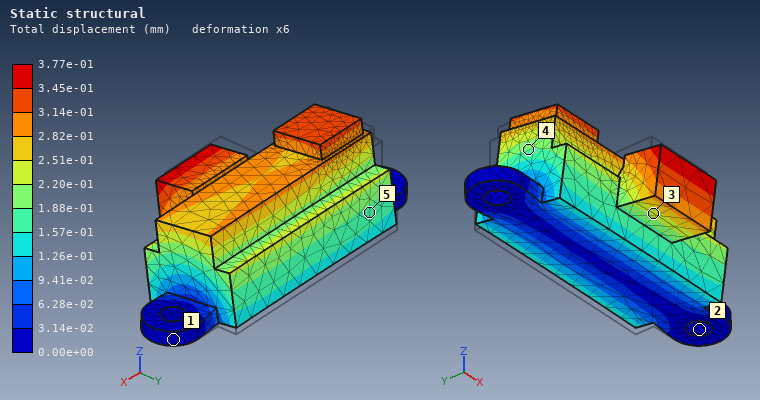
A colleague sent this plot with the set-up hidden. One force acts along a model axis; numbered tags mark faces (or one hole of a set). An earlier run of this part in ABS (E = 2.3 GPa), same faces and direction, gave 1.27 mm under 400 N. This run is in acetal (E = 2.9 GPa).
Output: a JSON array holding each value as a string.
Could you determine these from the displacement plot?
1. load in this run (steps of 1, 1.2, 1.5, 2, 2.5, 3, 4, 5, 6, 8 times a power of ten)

["150 N"]
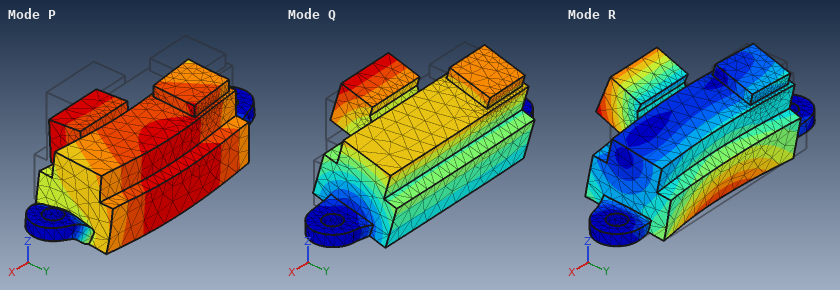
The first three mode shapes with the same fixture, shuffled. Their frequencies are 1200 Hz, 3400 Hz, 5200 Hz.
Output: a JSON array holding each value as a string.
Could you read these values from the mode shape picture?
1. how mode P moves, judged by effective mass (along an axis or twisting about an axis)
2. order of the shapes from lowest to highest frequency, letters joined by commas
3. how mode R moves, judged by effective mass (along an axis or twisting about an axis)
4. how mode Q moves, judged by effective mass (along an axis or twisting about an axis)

["along Z", "Q, P, R", "along Y", "along Y"]
